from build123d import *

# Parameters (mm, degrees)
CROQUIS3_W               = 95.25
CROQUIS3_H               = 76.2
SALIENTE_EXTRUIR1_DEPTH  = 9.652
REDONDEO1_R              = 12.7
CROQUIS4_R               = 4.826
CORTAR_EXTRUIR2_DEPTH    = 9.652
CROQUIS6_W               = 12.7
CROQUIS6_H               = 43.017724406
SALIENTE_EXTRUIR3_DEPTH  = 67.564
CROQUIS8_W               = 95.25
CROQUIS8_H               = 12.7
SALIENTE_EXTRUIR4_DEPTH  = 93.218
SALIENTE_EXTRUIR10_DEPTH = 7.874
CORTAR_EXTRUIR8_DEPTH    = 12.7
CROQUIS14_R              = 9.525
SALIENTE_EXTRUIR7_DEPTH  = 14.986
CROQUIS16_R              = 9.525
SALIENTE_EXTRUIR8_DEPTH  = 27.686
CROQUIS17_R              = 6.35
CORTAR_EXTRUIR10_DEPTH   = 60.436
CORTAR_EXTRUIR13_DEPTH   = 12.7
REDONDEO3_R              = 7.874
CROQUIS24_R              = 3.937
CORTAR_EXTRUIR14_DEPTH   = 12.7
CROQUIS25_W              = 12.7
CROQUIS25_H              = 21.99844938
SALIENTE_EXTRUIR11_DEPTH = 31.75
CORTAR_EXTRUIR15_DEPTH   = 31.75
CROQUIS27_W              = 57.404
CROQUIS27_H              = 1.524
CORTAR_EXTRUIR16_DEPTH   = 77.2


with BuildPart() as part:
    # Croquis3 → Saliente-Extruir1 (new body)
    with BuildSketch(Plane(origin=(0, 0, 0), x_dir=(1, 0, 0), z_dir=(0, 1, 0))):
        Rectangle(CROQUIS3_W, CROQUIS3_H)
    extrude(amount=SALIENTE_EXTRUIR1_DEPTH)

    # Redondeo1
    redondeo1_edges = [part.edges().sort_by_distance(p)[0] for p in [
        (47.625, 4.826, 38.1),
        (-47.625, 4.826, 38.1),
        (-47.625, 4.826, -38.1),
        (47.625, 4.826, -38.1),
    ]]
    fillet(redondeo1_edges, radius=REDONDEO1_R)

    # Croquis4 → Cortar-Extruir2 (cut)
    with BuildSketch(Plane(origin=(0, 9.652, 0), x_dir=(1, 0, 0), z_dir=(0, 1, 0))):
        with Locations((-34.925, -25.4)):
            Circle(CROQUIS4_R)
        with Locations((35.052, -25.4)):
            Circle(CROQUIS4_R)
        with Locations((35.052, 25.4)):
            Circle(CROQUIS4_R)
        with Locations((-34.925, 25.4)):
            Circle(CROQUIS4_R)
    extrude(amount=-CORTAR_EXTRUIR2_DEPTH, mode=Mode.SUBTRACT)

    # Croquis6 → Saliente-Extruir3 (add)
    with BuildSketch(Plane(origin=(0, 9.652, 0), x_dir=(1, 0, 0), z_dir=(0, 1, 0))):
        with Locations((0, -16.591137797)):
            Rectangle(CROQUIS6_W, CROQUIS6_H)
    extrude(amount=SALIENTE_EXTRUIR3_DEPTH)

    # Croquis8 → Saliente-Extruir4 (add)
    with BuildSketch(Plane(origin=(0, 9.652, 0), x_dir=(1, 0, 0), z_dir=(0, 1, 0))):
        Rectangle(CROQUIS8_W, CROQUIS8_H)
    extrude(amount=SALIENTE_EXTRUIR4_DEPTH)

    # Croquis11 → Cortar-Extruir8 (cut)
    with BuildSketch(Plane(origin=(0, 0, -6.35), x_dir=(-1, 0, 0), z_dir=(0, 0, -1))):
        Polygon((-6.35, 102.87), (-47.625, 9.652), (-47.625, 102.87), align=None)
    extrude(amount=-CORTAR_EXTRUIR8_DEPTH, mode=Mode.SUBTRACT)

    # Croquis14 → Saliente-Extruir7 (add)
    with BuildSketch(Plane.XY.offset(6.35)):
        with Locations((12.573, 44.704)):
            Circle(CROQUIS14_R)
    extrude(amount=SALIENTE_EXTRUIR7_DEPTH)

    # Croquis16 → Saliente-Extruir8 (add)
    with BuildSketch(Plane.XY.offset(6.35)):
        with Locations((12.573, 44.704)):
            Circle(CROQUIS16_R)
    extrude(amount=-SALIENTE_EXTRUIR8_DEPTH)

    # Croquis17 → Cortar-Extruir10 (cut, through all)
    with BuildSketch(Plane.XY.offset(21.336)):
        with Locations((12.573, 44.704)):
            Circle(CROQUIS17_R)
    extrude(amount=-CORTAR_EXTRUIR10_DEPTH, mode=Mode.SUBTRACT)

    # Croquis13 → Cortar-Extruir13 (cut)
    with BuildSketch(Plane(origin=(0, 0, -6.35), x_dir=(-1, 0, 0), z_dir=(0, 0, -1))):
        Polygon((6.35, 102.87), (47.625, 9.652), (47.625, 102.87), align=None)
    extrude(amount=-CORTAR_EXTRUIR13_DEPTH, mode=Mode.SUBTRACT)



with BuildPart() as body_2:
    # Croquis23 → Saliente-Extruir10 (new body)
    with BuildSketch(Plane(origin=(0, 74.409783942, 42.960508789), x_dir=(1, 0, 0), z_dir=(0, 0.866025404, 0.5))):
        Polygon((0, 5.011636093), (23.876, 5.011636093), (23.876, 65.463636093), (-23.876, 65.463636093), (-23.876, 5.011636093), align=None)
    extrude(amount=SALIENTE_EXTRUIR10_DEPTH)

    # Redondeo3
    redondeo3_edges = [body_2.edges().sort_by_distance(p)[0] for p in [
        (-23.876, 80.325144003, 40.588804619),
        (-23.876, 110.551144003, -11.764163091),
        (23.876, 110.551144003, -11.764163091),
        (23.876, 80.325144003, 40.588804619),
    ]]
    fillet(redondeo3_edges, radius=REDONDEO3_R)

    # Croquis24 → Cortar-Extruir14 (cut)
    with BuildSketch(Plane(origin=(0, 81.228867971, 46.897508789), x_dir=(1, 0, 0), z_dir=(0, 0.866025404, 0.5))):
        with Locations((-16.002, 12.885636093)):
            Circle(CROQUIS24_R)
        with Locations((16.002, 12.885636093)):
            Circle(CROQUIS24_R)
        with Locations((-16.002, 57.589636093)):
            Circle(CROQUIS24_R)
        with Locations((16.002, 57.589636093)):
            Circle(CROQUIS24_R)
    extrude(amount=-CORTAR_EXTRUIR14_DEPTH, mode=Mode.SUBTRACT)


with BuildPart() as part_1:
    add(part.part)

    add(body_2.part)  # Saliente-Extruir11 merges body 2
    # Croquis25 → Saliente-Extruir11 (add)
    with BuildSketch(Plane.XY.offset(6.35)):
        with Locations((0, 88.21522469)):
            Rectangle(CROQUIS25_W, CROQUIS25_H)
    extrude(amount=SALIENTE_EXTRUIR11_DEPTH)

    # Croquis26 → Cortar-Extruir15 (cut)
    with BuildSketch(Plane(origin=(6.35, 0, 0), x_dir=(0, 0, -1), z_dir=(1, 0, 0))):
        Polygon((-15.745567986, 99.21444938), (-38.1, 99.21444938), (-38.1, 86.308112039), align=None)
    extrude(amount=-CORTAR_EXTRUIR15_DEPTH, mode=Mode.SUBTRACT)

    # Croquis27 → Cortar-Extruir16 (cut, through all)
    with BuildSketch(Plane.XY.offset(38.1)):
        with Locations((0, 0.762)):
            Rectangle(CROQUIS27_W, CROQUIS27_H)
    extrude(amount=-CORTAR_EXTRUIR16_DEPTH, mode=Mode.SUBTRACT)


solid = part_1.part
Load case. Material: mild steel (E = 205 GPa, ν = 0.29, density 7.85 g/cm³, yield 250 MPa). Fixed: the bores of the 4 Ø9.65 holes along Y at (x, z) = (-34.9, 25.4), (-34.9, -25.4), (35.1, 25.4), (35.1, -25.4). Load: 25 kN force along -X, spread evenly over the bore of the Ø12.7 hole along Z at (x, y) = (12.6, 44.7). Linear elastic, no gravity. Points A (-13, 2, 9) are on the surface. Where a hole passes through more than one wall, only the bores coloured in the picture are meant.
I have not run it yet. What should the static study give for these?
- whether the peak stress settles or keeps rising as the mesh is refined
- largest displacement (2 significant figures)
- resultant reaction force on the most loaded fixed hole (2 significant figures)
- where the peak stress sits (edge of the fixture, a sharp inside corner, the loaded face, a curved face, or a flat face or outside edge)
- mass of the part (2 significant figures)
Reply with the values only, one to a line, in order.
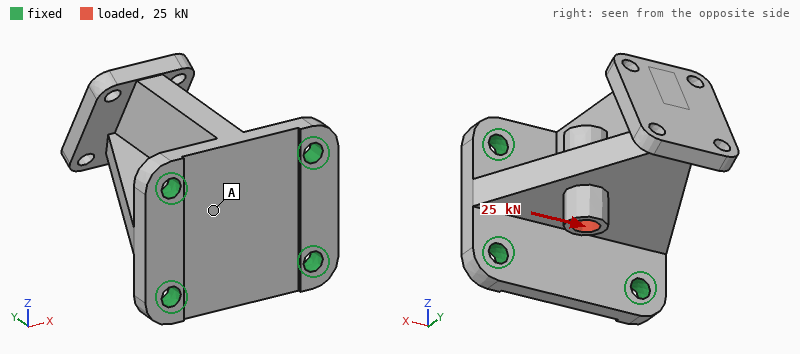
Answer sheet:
keeps rising
80 µm
11 kN
edge of the fixture
1.4 kg
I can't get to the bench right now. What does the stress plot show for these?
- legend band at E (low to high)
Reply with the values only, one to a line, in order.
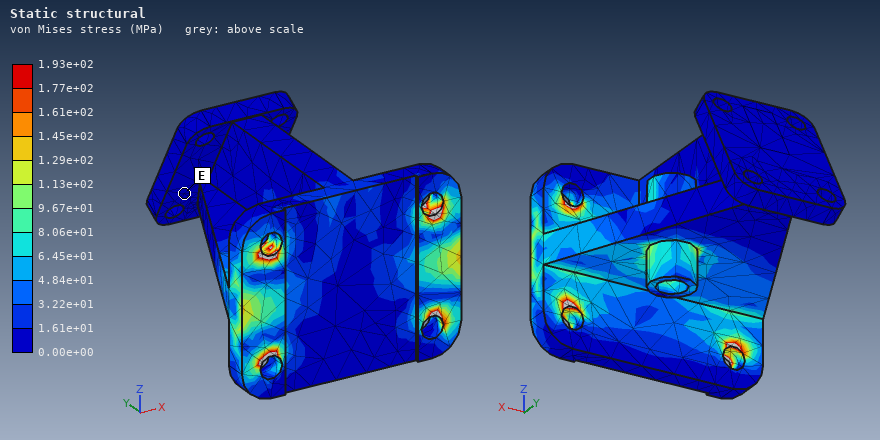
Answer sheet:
0.00e+00 to 1.61e+01 MPa
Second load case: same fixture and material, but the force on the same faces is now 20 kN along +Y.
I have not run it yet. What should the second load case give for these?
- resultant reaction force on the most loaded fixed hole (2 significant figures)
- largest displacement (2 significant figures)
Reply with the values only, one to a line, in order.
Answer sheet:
7.1 kN
47 µm
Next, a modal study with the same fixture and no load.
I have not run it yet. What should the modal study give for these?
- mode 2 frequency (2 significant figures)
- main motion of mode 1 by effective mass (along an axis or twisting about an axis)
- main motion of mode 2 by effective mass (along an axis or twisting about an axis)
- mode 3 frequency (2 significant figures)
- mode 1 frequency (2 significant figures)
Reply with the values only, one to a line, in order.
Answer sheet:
2700 Hz
along Z
along X
4200 Hz
1500 Hz
